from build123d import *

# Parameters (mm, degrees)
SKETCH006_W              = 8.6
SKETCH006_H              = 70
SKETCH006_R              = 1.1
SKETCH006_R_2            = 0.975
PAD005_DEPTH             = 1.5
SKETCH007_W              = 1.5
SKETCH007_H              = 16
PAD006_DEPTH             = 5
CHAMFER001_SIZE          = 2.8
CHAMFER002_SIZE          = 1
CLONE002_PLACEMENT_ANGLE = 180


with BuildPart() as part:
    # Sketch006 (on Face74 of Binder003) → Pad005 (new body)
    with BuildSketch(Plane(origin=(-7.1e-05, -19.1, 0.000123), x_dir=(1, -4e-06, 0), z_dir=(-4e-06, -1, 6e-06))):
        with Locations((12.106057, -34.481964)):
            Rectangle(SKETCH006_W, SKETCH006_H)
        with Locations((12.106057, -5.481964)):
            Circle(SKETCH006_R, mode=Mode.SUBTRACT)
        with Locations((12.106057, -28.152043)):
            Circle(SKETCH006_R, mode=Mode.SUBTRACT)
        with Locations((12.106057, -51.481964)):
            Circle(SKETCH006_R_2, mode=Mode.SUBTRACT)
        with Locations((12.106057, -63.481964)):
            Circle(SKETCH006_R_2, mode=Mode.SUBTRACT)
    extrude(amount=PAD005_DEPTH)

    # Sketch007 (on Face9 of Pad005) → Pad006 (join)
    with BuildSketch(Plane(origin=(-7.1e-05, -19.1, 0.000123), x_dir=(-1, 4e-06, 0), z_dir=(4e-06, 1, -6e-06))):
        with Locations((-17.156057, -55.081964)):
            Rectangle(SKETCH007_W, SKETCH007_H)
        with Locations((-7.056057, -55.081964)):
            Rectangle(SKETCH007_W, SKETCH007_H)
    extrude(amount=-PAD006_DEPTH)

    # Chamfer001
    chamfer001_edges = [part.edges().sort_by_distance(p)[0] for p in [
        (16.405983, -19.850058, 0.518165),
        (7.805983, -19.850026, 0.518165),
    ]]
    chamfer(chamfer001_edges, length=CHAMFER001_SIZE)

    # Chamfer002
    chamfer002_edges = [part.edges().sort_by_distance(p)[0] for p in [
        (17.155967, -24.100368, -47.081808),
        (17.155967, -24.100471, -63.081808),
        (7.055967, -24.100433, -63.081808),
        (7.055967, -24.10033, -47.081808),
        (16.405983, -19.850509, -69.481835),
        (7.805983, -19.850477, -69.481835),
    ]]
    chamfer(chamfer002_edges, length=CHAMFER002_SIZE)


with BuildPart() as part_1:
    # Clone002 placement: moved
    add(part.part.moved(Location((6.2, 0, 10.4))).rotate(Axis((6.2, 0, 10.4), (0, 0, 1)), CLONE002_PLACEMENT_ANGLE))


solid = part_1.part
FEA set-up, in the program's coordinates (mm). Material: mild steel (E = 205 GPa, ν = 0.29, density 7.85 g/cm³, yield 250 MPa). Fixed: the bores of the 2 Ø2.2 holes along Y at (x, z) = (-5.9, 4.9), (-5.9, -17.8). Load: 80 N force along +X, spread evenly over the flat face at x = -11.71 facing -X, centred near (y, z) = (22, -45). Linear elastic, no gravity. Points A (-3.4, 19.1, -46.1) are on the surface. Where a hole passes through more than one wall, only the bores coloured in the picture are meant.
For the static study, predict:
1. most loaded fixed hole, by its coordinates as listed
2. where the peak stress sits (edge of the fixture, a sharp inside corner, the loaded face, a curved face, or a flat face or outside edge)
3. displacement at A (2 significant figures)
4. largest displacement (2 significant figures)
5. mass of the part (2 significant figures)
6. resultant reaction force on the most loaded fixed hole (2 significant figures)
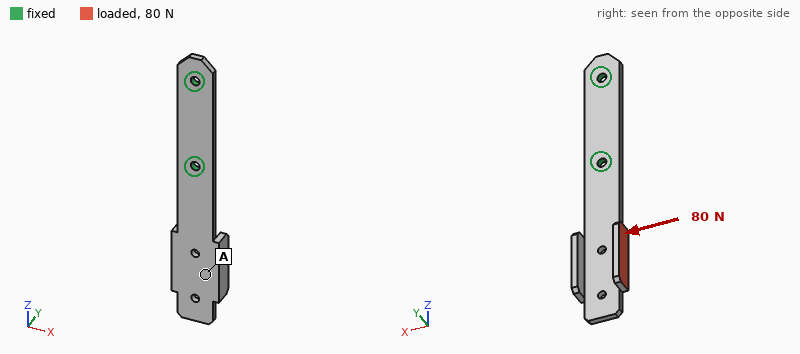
(-5.9, -17.8)
edge of the fixture
49 µm
89 µm
8.7 g
140 N
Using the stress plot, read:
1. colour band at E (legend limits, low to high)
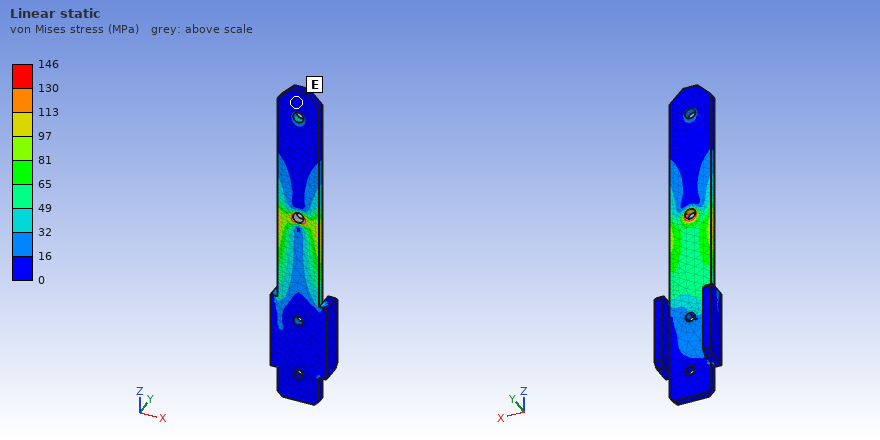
0 to 16 MPa
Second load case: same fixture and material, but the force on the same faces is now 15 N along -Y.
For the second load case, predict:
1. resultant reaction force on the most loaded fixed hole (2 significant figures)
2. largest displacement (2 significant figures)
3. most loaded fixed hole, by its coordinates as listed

16 N
0.34 mm
(-5.9, -17.8)
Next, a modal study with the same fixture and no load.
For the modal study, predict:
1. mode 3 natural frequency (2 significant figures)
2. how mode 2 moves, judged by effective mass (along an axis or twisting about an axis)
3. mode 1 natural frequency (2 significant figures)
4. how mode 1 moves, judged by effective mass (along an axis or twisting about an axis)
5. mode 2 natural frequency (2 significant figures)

3500 Hz
along X
620 Hz
along Y
2700 Hz
